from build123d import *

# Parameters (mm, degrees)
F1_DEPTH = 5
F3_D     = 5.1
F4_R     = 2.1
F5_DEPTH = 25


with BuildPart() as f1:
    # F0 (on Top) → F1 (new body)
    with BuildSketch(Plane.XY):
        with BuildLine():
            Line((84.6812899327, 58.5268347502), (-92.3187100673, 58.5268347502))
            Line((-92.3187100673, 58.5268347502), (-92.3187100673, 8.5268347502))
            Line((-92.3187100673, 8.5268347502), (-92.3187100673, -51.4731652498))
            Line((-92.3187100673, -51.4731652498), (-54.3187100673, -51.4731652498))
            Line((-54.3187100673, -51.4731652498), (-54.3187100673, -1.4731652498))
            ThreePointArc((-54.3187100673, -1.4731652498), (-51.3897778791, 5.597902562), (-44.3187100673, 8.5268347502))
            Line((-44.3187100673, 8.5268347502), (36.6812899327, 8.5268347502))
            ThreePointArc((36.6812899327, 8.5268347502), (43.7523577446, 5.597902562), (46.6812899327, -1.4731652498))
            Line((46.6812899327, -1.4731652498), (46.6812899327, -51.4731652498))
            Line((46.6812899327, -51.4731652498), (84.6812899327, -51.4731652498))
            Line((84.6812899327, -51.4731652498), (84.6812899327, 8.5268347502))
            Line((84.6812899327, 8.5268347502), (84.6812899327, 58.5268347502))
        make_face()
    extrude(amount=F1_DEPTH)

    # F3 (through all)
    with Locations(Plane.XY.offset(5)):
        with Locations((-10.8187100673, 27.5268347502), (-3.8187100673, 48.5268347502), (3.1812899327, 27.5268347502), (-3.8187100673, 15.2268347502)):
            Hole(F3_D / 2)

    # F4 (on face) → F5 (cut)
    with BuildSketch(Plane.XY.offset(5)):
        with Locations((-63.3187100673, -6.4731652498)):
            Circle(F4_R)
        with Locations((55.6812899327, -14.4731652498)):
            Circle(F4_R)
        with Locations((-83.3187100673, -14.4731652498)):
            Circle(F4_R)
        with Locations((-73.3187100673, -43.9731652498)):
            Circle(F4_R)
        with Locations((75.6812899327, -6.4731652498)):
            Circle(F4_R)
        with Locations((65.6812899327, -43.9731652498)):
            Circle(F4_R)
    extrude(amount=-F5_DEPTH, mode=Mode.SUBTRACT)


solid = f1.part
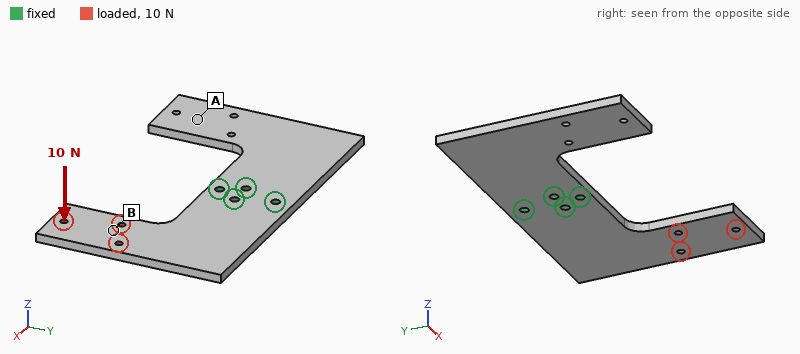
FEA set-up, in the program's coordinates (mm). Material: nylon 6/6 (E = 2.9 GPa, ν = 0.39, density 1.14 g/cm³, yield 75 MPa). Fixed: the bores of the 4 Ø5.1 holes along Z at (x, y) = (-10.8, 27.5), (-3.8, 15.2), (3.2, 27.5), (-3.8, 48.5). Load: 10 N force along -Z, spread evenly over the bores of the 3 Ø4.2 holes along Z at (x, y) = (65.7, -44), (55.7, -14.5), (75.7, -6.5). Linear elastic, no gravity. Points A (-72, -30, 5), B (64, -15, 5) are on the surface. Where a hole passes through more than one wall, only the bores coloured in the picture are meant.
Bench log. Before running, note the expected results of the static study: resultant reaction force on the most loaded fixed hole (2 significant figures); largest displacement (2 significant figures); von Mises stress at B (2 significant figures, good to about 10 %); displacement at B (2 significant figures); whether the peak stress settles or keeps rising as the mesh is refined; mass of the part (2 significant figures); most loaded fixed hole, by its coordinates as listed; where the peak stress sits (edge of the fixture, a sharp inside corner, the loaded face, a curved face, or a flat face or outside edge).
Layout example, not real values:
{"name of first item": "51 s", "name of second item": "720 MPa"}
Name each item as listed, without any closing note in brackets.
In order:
{"resultant reaction force on the most loaded fixed hole": "35 N", "largest displacement": "2.2 mm", "von Mises stress at B": "0.77 MPa", "displacement at B": "1.2 mm", "whether the peak stress settles or keeps rising as the mesh is refined": "keeps rising", "mass of the part": "76 g", "most loaded fixed hole, by its coordinates as listed": "(3.2, 27.5)", "where the peak stress sits": "edge of the fixture"}
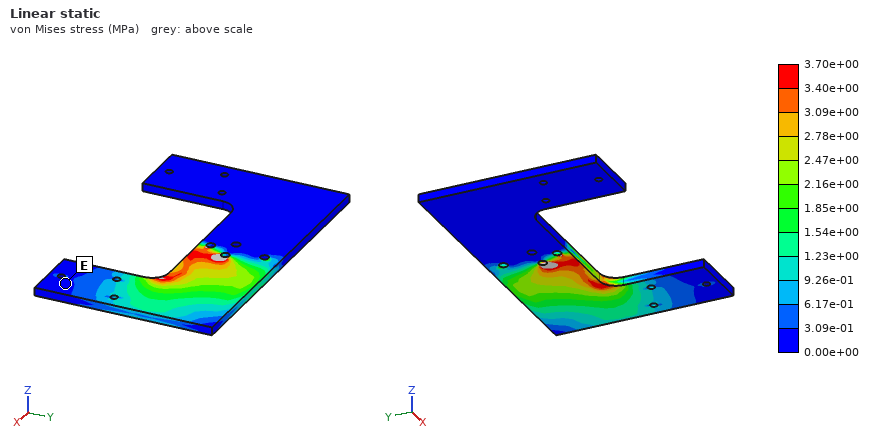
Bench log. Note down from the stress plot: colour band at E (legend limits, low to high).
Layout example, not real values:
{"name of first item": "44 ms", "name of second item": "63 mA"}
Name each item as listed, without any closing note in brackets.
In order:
{"colour band at E": "0.00e+00 to 3.09e-01 MPa"}
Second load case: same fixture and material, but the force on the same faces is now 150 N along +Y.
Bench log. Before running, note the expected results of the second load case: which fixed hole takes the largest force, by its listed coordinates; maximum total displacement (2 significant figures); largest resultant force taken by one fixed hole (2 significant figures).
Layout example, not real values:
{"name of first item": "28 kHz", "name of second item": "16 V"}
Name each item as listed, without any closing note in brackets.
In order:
{"which fixed hole takes the largest force, by its listed coordinates": "(-3.8, 48.5)", "maximum total displacement": "0.32 mm", "largest resultant force taken by one fixed hole": "280 N"}
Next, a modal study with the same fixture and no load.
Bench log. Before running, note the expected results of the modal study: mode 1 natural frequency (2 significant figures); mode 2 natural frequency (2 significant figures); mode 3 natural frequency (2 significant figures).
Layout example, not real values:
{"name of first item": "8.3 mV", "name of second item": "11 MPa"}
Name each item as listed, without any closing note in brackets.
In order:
{"mode 1 natural frequency": "110 Hz", "mode 2 natural frequency": "110 Hz", "mode 3 natural frequency": "220 Hz"}
